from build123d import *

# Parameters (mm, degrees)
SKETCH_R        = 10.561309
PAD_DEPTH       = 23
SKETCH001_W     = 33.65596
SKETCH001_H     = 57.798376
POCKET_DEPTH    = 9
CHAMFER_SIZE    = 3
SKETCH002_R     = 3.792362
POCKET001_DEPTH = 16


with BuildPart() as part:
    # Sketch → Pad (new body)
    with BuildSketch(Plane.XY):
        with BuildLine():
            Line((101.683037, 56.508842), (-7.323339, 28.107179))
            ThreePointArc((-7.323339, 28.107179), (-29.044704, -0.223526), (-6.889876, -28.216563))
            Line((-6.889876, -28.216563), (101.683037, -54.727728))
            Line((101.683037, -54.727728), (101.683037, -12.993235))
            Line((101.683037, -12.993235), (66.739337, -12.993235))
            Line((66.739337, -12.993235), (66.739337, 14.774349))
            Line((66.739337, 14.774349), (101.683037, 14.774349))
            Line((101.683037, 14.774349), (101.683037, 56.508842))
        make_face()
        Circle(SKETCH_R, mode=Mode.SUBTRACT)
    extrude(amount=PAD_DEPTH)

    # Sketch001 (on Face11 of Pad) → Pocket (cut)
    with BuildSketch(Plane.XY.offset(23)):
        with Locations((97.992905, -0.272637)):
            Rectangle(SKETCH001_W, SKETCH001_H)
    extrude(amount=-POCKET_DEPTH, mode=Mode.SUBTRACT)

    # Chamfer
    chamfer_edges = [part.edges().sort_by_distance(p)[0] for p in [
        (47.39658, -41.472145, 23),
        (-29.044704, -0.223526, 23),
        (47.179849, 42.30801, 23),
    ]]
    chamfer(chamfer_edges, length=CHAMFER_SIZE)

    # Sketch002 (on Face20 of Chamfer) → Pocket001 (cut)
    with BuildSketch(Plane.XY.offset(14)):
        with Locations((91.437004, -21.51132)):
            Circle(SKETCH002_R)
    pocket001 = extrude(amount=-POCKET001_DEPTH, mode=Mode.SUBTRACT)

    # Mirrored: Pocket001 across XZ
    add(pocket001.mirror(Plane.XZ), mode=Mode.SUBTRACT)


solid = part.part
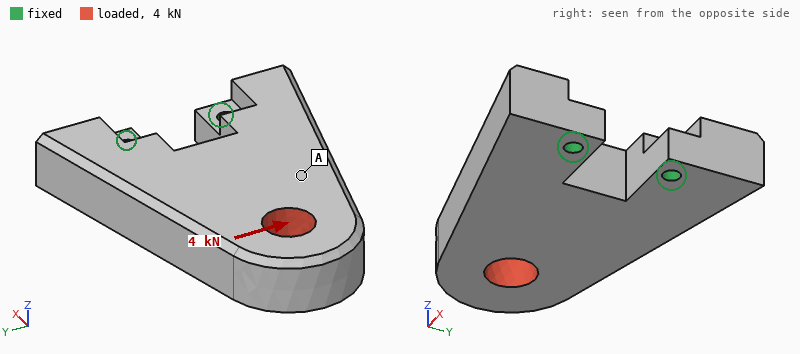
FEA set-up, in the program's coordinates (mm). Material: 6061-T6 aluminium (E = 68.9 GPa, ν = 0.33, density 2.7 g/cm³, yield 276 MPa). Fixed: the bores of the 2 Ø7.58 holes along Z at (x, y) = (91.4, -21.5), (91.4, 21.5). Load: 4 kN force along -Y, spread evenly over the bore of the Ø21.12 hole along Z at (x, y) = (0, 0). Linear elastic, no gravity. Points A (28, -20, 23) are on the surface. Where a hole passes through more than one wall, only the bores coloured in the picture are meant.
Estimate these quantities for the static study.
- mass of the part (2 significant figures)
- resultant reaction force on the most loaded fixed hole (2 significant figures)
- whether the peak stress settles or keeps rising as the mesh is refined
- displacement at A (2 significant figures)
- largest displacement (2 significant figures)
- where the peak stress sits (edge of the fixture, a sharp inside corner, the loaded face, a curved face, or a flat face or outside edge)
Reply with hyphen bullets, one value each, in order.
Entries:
- 520 g
- 6.6 kN
- keeps rising
- 46 µm
- 83 µm
- edge of the fixture
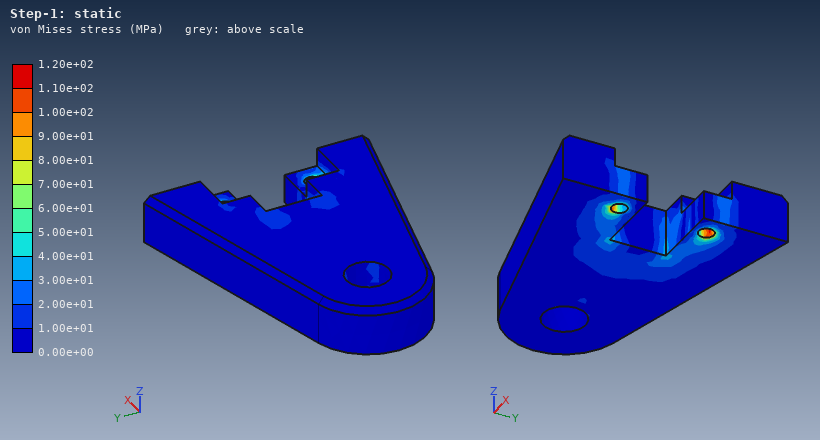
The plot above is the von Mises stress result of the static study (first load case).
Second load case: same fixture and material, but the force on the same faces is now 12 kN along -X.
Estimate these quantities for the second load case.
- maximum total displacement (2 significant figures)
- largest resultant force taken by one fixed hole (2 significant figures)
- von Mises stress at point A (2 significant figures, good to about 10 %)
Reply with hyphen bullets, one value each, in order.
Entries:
- 83 µm
- 6.1 kN
- 8.0 MPa
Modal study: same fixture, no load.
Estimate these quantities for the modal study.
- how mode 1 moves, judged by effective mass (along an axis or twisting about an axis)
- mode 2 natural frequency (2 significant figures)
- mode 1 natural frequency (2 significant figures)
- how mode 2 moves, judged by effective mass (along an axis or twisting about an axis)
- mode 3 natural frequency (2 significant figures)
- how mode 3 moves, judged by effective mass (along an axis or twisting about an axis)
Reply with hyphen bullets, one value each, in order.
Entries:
- along Z
- 2500 Hz
- 970 Hz
- along Y
- 3700 Hz
- twisting about X
